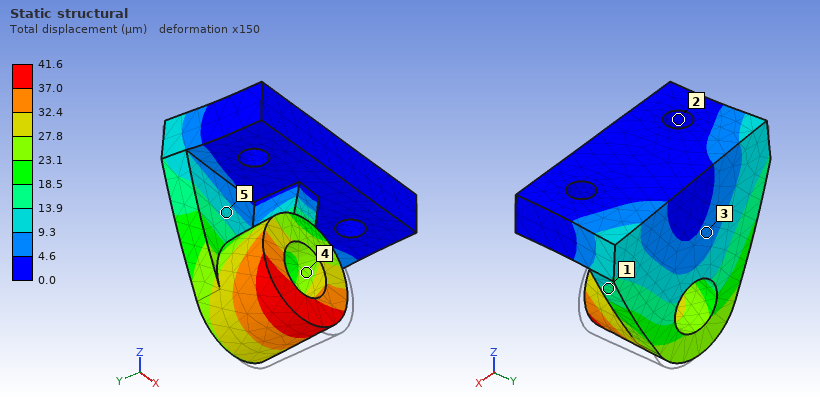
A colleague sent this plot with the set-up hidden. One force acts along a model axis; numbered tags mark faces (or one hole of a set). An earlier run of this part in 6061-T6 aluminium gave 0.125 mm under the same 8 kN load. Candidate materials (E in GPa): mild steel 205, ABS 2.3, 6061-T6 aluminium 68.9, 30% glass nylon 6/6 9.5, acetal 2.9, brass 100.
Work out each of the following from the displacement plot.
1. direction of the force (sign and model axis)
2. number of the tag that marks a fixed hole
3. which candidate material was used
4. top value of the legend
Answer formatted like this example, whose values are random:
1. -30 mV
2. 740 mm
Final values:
1. -X
2. 2
3. mild steel
4. 41.6 µm
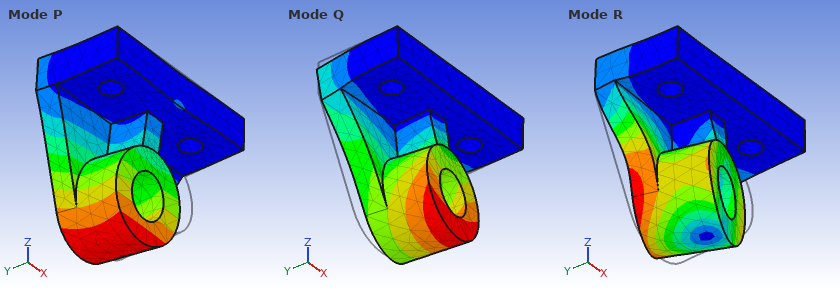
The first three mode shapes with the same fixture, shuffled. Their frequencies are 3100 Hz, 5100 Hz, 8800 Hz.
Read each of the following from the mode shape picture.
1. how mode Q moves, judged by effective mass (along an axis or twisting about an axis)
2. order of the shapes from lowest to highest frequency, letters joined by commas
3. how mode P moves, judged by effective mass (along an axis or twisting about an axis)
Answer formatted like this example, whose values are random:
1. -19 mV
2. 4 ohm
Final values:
1. along X
2. P, Q, R
3. along Y
